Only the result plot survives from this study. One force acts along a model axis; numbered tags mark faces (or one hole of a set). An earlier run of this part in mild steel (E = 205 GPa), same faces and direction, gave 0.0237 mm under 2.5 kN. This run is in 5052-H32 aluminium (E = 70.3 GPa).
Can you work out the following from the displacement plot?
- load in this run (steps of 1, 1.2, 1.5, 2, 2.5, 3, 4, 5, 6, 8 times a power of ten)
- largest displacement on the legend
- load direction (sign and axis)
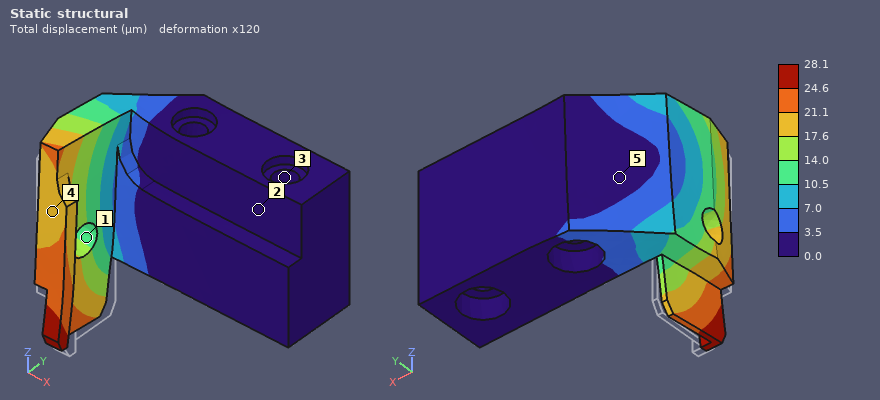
1 kN
28.1 µm
+Z
